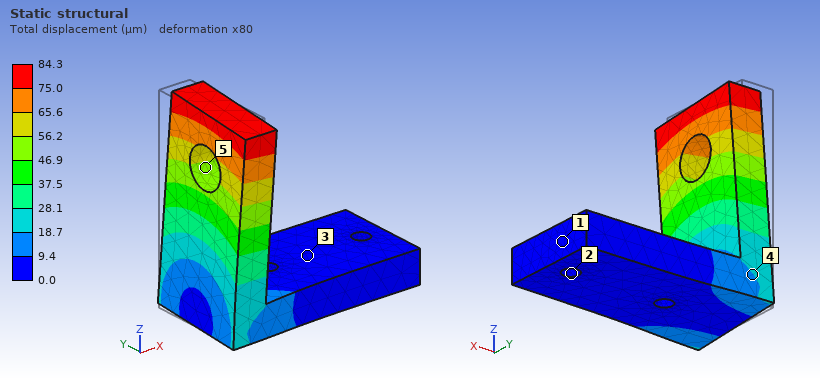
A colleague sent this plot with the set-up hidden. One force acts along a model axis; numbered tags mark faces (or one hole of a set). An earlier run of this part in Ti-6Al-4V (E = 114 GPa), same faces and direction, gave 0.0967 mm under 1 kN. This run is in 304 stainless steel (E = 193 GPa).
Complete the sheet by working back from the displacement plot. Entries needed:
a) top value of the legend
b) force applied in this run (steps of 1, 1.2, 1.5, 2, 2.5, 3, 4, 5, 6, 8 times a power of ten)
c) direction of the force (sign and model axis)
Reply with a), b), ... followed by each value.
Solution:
a) 84.3 µm
b) 1.5 kN
c) -Y
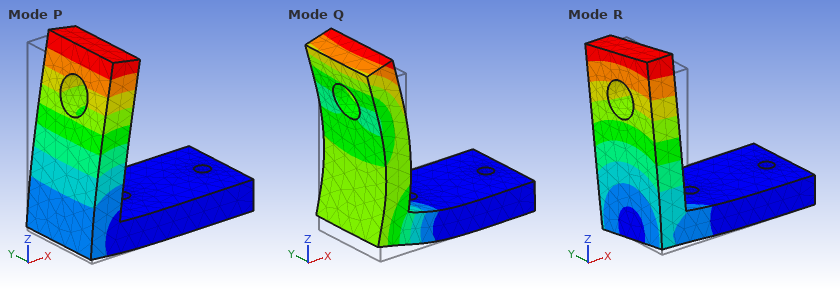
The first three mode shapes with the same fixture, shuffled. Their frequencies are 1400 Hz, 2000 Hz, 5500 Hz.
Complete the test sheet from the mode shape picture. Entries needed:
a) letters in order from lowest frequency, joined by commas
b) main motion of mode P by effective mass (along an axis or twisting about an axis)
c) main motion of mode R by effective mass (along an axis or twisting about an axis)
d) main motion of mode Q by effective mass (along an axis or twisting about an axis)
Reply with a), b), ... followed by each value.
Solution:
a) P, R, Q
b) along X
c) along Y
d) along Z
